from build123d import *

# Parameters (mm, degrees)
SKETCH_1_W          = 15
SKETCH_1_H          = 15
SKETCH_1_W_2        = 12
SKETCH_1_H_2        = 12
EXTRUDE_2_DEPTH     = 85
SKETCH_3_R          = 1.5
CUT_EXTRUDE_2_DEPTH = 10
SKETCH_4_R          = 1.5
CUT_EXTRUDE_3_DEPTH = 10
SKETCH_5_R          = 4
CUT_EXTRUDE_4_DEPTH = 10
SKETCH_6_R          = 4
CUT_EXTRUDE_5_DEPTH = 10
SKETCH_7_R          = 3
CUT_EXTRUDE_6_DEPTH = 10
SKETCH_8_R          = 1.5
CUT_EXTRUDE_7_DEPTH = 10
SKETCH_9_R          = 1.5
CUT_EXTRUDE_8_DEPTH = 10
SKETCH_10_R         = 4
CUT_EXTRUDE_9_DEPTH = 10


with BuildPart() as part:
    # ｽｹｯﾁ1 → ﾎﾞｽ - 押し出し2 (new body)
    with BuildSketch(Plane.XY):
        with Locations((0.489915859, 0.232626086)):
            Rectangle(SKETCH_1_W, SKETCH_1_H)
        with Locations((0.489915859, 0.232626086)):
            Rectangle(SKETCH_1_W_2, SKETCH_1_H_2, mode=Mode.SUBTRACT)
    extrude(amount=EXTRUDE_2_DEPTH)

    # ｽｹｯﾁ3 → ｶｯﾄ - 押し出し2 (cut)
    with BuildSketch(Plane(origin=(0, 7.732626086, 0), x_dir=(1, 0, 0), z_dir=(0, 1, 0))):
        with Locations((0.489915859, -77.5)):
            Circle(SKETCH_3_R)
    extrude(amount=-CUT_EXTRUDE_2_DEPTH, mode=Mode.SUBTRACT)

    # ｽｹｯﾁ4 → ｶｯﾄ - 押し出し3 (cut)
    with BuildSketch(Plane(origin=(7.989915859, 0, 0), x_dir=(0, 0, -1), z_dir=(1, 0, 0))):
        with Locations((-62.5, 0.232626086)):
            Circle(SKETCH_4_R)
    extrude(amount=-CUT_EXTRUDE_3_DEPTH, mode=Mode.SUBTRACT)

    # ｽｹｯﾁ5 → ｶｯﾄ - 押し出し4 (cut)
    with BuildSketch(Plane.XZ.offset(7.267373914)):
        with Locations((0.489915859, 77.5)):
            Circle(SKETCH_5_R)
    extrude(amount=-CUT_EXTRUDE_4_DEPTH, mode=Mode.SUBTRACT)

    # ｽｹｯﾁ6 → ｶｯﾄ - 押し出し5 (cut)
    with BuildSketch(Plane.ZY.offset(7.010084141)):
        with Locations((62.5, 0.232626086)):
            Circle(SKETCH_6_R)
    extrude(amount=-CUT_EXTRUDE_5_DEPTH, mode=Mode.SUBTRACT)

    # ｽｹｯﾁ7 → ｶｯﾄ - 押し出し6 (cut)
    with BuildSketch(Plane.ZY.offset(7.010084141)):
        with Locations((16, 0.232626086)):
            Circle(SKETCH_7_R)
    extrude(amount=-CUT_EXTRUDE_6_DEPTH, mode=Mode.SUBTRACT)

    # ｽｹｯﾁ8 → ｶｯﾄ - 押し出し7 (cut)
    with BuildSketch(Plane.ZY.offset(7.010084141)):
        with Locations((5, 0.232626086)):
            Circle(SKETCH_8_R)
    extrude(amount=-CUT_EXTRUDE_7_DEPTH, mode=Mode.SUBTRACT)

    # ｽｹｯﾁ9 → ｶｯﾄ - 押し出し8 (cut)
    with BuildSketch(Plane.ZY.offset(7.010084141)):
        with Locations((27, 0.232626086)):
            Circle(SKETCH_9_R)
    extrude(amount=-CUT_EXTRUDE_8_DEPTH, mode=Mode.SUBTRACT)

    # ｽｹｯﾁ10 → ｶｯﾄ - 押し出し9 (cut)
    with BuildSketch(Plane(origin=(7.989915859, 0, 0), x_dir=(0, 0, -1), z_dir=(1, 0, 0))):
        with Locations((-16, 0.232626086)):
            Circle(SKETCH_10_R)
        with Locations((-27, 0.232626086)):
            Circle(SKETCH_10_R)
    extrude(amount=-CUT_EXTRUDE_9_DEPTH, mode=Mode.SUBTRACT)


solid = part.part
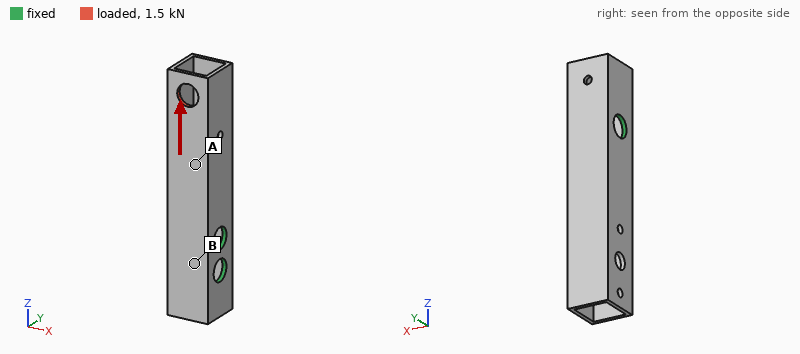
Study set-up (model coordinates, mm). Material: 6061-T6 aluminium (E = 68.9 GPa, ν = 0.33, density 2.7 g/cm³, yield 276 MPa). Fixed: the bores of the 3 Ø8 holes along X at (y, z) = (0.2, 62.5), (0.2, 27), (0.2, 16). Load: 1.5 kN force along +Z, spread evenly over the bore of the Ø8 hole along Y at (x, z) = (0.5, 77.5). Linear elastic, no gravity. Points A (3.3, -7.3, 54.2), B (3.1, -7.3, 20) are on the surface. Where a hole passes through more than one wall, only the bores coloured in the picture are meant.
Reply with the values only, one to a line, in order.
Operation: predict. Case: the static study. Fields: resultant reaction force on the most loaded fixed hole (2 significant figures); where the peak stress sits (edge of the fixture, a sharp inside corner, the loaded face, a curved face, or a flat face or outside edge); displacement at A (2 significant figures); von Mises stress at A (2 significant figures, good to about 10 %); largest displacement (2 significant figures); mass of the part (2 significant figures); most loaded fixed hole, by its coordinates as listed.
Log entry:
950 N
the loaded face
14 µm
32 MPa
61 µm
18 g
(0.2, 62.5)
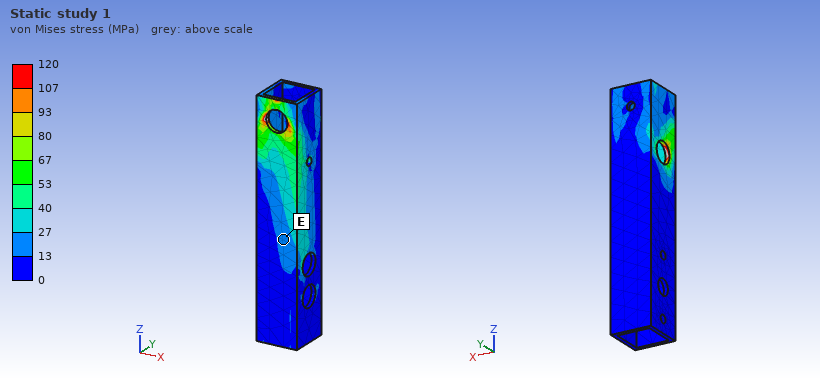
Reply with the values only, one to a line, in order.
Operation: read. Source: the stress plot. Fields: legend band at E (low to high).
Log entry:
13 to 27 MPa
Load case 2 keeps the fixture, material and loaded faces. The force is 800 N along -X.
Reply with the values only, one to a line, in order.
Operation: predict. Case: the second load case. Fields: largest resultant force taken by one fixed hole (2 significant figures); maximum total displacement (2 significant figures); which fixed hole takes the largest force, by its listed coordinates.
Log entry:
1.1 kN
0.11 mm
(0.2, 62.5)
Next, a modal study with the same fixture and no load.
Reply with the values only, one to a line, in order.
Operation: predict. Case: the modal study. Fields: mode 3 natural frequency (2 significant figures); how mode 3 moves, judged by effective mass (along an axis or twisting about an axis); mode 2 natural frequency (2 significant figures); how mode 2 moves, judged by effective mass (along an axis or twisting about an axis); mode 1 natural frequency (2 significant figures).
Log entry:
11 kHz
along X
9300 Hz
along Y
6000 Hz
